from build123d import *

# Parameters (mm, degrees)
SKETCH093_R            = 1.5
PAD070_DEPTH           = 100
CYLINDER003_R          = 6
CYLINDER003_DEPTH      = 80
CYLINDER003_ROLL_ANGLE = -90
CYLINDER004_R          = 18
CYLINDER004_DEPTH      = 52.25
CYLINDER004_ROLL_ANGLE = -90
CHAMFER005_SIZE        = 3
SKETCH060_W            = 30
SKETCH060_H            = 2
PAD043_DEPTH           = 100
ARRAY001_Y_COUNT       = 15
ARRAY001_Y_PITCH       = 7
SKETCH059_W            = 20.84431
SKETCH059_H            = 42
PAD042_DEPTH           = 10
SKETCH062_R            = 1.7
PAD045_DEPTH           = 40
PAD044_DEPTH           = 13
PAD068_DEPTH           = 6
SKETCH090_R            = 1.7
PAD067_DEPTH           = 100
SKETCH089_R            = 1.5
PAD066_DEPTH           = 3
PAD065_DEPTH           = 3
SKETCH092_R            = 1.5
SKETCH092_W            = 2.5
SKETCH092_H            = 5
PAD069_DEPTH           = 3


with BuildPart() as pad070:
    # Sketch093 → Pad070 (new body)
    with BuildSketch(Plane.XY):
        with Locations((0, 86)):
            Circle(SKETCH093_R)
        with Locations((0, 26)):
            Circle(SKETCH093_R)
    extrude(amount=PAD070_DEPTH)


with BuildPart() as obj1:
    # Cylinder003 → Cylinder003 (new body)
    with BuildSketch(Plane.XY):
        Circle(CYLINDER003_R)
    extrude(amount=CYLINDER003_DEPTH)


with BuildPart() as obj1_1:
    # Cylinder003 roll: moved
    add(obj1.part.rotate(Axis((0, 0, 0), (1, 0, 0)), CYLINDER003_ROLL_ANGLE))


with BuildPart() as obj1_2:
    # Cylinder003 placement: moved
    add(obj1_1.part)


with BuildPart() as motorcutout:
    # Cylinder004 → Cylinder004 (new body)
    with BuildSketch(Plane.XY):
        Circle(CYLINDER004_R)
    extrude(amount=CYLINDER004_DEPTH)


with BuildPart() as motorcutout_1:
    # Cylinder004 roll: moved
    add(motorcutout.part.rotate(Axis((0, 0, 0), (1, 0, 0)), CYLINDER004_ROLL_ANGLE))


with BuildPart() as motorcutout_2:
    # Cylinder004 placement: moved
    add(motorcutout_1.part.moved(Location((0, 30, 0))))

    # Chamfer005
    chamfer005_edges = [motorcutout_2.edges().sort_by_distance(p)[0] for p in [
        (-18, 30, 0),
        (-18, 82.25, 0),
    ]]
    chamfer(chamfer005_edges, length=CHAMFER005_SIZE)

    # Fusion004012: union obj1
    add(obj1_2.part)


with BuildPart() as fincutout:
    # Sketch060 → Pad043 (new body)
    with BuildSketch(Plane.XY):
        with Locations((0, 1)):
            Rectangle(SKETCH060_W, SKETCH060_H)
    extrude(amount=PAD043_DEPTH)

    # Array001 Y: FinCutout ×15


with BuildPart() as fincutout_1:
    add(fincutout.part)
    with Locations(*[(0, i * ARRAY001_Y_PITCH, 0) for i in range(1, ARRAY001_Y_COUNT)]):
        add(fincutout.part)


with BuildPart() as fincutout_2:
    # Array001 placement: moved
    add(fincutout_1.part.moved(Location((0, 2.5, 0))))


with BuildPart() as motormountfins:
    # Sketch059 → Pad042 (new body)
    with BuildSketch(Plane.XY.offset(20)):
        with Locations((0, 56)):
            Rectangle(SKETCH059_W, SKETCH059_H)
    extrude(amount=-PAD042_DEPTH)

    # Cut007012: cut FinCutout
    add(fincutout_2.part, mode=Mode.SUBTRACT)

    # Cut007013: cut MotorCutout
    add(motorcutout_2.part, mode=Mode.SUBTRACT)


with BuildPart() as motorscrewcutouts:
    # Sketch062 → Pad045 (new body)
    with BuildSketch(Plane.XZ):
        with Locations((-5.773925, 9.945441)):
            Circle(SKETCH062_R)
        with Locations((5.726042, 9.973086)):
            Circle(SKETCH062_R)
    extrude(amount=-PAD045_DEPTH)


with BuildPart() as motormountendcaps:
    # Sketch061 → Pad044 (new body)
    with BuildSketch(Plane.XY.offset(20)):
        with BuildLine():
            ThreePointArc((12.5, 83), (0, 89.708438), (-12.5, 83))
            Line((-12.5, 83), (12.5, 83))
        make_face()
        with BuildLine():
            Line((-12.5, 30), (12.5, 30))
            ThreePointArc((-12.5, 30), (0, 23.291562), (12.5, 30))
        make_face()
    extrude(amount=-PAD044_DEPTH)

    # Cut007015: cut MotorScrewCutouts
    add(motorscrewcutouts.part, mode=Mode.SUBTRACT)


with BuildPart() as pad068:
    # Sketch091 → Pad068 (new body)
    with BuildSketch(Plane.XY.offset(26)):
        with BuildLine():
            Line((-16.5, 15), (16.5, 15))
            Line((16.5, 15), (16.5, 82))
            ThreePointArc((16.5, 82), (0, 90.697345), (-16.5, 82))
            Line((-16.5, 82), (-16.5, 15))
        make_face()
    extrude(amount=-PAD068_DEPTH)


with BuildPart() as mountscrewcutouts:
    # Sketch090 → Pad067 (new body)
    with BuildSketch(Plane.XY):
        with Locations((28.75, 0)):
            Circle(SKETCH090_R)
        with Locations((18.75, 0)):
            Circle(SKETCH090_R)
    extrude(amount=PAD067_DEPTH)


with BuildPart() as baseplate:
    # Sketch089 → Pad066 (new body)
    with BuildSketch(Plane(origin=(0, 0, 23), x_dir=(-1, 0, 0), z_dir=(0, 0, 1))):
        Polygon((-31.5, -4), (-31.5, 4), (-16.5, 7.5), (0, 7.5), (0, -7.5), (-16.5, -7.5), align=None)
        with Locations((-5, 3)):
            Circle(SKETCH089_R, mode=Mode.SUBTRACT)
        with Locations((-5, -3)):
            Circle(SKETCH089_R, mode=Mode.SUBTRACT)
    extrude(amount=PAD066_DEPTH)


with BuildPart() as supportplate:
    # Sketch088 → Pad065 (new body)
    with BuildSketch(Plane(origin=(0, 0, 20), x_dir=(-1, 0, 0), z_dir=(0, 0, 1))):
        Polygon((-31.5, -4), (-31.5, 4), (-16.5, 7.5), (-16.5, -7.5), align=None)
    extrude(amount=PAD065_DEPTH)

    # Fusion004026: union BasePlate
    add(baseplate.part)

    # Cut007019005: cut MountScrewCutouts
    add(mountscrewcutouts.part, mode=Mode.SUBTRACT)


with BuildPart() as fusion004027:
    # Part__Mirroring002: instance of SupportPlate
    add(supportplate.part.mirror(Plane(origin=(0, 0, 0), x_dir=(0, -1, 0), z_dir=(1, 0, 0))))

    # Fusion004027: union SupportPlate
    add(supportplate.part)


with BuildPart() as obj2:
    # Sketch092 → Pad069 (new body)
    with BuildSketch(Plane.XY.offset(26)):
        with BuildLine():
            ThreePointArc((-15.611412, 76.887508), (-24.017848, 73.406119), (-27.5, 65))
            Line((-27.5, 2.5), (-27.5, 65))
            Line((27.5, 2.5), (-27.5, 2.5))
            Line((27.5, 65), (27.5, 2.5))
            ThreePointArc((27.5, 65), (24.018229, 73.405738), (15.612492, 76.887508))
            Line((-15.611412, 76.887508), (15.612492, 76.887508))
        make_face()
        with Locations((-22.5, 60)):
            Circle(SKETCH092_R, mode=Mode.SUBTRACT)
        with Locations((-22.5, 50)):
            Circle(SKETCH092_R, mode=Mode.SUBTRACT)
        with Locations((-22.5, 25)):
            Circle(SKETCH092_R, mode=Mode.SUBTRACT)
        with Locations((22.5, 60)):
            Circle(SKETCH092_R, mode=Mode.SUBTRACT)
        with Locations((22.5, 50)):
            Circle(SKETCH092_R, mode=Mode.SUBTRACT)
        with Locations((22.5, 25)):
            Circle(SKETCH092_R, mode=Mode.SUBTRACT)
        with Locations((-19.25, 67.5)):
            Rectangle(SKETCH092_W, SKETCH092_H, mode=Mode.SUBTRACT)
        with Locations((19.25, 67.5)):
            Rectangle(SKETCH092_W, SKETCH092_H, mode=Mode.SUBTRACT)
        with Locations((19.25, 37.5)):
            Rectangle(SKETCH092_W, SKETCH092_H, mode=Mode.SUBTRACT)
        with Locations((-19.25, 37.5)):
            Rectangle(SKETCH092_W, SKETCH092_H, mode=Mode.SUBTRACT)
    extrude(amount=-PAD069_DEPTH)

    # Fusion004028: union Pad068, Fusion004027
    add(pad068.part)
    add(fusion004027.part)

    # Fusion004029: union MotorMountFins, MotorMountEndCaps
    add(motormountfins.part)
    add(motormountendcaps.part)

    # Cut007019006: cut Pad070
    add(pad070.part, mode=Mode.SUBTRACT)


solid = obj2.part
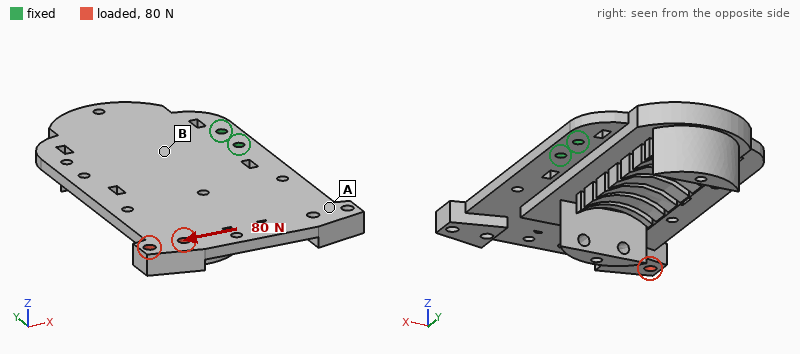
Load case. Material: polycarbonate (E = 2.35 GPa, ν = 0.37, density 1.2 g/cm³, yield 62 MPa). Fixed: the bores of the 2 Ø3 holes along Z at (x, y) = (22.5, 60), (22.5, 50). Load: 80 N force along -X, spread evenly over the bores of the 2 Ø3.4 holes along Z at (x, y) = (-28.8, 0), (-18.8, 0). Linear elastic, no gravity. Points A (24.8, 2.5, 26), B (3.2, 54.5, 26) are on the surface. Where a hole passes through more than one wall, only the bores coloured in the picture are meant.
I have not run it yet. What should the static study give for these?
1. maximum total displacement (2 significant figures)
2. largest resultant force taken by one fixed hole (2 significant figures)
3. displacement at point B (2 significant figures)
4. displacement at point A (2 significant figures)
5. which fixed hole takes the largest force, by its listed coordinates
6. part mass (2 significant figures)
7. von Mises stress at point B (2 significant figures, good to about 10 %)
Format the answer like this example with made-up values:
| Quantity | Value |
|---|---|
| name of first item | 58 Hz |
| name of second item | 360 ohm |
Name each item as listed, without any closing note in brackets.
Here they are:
| Quantity | Value |
|---|---|
| maximum total displacement | 1.1 mm |
| largest resultant force taken by one fixed hole | 390 N |
| displacement at point B | 0.19 mm |
| displacement at point A | 0.54 mm |
| which fixed hole takes the largest force, by its listed coordinates | (22.5, 50) |
| part mass | 33 g |
| von Mises stress at point B | 2.9 MPa |
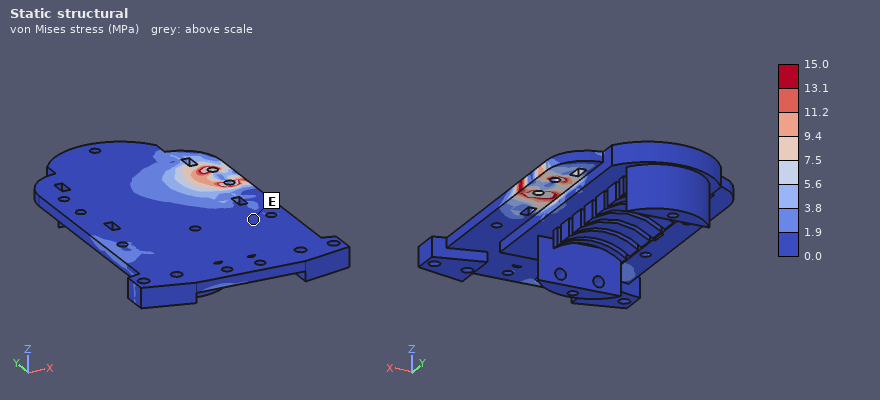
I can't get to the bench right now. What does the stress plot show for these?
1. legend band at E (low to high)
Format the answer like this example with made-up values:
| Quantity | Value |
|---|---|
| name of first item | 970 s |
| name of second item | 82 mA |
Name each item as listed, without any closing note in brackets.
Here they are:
| Quantity | Value |
|---|---|
| legend band at E | 0.0 to 1.9 MPa |
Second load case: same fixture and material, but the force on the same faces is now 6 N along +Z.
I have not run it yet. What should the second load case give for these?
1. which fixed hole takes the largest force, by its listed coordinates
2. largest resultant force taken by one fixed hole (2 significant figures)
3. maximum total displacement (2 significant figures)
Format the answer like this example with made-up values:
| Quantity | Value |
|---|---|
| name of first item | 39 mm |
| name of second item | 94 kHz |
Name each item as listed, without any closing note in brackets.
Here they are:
| Quantity | Value |
|---|---|
| which fixed hole takes the largest force, by its listed coordinates | (22.5, 50) |
| largest resultant force taken by one fixed hole | 24 N |
| maximum total displacement | 1.3 mm |
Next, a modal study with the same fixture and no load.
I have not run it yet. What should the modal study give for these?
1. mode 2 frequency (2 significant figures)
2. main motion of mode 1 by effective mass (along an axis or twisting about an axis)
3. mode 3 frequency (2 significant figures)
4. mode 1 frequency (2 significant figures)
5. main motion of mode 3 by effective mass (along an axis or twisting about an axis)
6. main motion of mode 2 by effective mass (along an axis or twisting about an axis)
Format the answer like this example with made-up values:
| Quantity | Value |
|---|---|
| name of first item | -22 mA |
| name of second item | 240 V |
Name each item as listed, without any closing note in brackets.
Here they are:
| Quantity | Value |
|---|---|
| mode 2 frequency | 260 Hz |
| main motion of mode 1 by effective mass | along Z |
| mode 3 frequency | 500 Hz |
| mode 1 frequency | 160 Hz |
| main motion of mode 3 by effective mass | along Y |
| main motion of mode 2 by effective mass | twisting about X |
